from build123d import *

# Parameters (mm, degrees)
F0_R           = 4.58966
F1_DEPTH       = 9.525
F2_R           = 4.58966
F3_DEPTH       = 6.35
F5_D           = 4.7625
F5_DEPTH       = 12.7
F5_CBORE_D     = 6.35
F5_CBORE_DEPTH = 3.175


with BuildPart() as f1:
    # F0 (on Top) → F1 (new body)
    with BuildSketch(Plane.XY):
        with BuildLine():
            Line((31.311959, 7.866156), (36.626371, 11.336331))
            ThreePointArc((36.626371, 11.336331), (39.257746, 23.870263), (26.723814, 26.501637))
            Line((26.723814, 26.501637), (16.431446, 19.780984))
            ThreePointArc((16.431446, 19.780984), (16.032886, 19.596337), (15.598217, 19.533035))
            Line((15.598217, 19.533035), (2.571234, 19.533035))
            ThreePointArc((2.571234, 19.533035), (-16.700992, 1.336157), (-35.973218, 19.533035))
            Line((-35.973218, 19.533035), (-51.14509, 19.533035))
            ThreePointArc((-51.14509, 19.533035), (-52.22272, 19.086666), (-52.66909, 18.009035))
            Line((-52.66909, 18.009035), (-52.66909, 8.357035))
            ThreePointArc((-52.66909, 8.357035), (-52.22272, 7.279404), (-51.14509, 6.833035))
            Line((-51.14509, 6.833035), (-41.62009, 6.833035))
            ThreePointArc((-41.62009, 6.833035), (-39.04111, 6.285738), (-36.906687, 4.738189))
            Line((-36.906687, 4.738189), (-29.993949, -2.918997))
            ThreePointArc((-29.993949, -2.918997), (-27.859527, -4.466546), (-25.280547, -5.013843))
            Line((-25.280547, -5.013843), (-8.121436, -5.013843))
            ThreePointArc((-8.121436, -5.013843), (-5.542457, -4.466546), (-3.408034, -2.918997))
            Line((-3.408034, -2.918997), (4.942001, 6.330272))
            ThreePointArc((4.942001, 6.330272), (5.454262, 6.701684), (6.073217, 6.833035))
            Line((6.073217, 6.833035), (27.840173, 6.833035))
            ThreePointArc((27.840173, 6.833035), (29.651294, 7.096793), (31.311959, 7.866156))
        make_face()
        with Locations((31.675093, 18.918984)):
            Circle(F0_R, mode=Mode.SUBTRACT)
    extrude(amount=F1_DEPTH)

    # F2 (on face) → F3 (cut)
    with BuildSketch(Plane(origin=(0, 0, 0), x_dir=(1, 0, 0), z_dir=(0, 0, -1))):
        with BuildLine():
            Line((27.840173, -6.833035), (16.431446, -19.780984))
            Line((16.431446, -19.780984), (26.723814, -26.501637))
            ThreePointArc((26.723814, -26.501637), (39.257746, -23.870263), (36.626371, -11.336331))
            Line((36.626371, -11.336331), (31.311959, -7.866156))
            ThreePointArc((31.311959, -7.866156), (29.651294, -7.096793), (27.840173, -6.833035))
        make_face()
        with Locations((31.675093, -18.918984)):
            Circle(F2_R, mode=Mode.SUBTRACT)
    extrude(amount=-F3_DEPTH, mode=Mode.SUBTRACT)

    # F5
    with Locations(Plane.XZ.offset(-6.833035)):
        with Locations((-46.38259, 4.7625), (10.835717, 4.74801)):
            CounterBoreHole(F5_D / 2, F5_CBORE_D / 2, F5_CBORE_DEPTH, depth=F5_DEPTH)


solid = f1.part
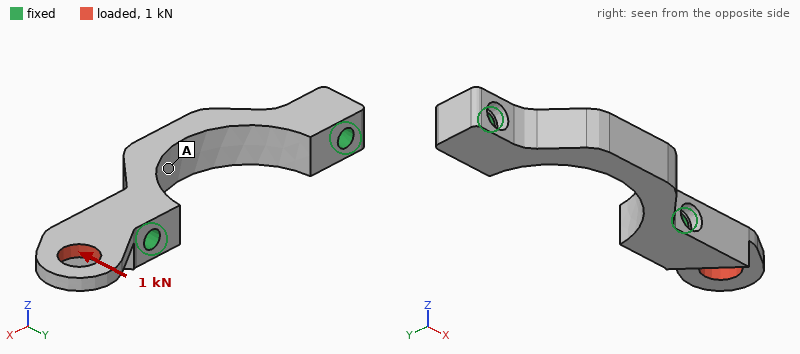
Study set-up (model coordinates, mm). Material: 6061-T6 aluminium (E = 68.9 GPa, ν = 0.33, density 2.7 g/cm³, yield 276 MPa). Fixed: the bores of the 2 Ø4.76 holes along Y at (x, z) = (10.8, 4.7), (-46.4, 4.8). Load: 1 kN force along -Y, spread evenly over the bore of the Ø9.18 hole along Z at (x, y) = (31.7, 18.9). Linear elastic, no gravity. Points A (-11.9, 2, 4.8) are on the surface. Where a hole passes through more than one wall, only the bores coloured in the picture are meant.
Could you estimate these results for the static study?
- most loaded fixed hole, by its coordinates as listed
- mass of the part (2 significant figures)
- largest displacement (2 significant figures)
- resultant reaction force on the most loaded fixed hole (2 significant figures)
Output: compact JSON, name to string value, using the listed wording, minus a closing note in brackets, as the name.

{"most loaded fixed hole, by its coordinates as listed": "(10.8, 4.7)", "mass of the part": "21 g", "largest displacement": "0.11 mm", "resultant reaction force on the most loaded fixed hole": "1.0 kN"}
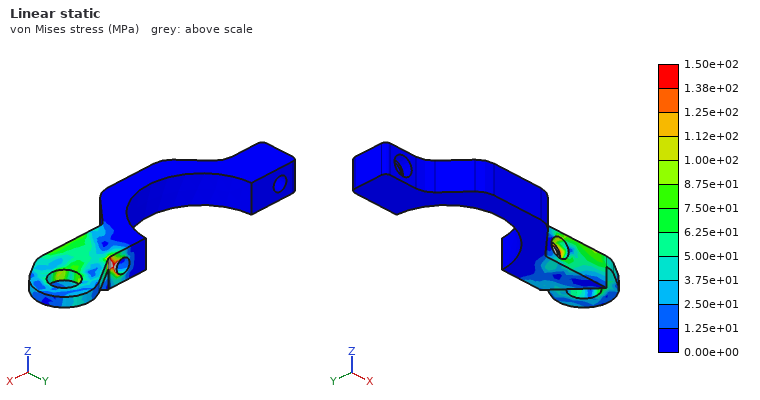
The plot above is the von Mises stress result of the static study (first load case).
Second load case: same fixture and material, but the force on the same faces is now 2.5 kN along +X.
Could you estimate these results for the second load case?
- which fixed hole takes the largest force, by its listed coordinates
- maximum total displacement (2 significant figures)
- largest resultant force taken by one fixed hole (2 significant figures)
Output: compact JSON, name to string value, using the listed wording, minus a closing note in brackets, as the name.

{"which fixed hole takes the largest force, by its listed coordinates": "(10.8, 4.7)", "maximum total displacement": "0.10 mm", "largest resultant force taken by one fixed hole": "2.5 kN"}
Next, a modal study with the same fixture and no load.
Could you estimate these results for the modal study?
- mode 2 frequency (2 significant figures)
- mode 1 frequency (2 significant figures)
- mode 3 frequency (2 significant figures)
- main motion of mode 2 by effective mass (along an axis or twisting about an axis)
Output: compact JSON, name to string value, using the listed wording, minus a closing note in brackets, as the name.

{"mode 2 frequency": "8500 Hz", "mode 1 frequency": "5900 Hz", "mode 3 frequency": "12 kHz", "main motion of mode 2 by effective mass": "along Z"}
